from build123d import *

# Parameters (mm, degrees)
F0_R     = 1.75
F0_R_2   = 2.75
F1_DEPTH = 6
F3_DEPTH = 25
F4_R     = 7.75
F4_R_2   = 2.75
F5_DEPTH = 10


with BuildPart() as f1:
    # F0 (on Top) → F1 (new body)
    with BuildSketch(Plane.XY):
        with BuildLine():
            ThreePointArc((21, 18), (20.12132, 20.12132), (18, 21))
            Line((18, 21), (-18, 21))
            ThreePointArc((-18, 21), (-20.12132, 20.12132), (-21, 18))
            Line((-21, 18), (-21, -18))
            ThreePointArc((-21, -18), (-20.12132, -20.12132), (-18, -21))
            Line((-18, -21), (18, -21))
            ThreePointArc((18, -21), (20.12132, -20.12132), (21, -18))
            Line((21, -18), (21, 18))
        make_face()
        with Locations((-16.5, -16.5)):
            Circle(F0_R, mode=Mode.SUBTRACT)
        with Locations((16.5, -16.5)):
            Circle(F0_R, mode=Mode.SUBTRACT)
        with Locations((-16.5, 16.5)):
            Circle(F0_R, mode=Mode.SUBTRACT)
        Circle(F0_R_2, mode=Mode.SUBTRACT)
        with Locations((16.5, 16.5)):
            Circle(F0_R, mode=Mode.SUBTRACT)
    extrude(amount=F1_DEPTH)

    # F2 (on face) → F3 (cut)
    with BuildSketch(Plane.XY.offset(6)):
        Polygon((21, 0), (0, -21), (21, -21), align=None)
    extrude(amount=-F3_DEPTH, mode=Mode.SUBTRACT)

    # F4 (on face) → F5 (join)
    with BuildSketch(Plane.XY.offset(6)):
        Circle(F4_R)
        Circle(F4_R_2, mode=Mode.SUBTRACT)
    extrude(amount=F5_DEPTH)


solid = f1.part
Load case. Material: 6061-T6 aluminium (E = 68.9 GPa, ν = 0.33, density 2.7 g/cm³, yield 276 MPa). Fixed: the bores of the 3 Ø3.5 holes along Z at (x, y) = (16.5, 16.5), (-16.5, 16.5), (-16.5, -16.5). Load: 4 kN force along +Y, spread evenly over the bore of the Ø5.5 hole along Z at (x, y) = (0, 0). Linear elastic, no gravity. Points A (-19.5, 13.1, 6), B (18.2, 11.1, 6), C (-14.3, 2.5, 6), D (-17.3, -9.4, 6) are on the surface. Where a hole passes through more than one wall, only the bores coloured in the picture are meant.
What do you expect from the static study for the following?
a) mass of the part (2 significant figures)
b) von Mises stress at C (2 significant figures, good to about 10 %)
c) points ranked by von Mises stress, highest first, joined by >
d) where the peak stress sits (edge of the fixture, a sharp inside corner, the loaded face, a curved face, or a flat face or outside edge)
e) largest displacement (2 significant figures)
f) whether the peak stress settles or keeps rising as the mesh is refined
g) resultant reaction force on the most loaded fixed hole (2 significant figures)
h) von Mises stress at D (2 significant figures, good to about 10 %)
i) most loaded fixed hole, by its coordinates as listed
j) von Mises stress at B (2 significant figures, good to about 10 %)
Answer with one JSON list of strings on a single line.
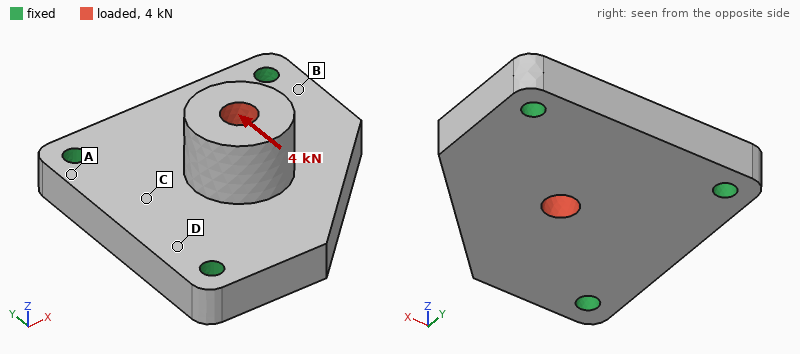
["29 g", "32 MPa", "B > C > D > A", "edge of the fixture", "43 µm", "keeps rising", "1.7 kN", "21 MPa", "(-16.5, 16.5)", "43 MPa"]
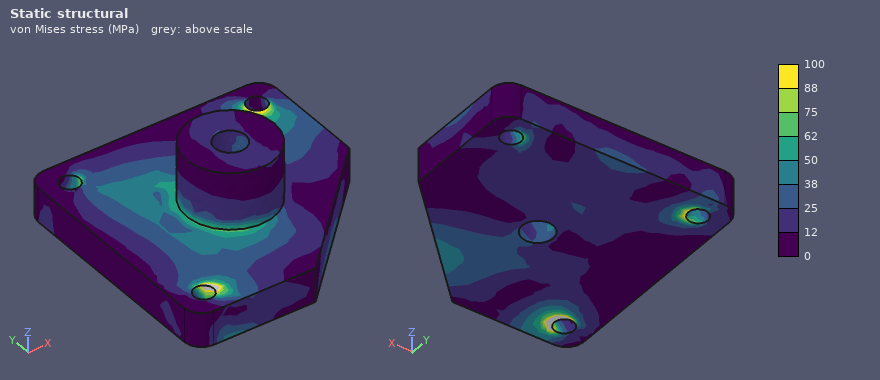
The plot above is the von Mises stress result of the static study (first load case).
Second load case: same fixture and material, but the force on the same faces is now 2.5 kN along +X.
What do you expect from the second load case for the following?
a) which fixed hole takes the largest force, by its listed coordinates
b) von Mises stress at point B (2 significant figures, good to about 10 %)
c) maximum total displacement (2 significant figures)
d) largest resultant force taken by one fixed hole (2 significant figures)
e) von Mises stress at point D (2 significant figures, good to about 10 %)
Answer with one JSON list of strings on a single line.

["(-16.5, 16.5)", "22 MPa", "27 µm", "1.1 kN", "11 MPa"]
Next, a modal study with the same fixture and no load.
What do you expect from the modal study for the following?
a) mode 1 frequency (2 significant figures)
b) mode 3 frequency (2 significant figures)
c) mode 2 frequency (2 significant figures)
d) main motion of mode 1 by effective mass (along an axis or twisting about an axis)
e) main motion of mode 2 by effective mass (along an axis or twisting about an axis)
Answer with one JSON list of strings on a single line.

["9300 Hz", "21 kHz", "18 kHz", "along Z", "along Z"]
